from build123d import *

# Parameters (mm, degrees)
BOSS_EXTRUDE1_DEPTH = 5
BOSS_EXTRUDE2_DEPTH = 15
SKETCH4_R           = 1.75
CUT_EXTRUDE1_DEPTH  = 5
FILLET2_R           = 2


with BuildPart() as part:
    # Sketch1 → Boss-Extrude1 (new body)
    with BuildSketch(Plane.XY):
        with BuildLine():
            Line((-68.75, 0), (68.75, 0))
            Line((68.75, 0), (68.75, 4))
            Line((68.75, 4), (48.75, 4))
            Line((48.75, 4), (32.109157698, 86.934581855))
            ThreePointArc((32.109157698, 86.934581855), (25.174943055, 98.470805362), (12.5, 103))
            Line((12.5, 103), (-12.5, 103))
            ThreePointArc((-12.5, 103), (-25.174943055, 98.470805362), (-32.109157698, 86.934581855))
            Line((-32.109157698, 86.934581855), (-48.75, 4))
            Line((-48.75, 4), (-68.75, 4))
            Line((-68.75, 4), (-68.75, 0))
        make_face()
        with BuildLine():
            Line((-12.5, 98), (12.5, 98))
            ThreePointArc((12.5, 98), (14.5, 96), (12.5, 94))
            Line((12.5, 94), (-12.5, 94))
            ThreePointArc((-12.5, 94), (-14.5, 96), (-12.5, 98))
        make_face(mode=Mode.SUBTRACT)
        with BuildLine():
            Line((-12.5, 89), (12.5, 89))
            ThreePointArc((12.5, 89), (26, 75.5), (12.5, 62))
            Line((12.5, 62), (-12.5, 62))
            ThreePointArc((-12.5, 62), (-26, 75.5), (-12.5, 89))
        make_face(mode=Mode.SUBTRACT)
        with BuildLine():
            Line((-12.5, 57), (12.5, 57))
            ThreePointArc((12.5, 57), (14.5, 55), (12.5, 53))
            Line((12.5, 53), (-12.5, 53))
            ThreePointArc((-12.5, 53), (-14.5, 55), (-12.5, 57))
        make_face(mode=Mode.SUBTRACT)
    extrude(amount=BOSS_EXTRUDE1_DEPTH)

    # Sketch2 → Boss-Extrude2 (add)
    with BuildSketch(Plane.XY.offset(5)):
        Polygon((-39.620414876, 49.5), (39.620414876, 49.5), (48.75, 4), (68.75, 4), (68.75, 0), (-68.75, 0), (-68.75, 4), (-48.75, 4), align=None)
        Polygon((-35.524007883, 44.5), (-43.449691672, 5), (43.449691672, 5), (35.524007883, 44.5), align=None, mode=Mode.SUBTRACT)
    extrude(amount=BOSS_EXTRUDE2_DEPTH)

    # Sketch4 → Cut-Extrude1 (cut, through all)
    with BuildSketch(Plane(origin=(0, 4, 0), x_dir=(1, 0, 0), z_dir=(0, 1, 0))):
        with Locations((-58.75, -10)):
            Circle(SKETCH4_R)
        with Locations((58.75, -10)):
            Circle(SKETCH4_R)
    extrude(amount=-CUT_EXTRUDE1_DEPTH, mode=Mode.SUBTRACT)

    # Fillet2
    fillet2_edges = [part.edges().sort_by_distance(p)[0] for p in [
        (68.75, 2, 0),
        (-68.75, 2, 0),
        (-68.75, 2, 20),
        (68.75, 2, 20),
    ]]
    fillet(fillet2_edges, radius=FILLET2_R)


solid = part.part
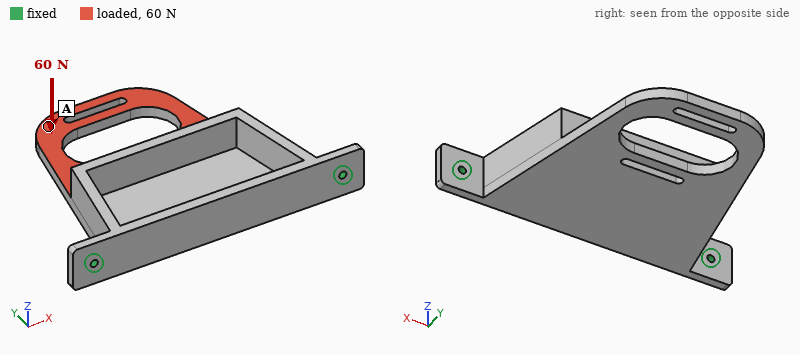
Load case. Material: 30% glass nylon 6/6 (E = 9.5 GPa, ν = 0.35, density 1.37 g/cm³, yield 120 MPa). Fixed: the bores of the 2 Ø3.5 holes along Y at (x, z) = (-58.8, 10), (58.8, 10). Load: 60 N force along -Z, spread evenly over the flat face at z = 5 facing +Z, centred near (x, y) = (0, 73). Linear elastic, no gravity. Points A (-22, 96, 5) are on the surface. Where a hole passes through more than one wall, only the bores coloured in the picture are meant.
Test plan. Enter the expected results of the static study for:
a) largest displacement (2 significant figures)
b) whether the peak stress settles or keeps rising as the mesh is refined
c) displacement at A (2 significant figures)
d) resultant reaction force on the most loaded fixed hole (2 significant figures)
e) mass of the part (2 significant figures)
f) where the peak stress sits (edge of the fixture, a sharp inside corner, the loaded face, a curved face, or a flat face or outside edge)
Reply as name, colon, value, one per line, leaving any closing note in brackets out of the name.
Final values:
largest displacement: 1.9 mm
whether the peak stress settles or keeps rising as the mesh is refined: keeps rising
displacement at A: 1.7 mm
resultant reaction force on the most loaded fixed hole: 31 N
mass of the part: 75 g
where the peak stress sits: edge of the fixture
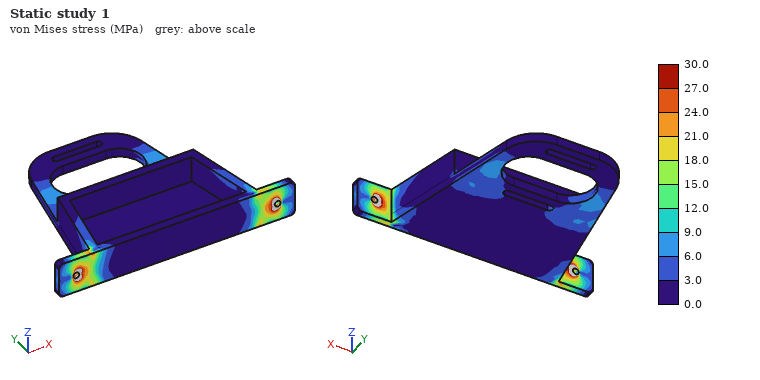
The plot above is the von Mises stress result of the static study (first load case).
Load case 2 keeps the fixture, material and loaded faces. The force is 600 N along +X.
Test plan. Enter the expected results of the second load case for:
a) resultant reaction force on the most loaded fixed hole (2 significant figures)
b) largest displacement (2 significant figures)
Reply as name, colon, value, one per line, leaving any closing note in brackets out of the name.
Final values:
resultant reaction force on the most loaded fixed hole: 500 N
largest displacement: 0.62 mm
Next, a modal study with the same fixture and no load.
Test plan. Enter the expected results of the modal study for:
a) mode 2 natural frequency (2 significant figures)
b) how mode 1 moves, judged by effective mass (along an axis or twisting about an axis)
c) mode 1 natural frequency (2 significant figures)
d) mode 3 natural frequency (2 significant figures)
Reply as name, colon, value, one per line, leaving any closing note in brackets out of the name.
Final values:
mode 2 natural frequency: 820 Hz
how mode 1 moves, judged by effective mass: along Z
mode 1 natural frequency: 230 Hz
mode 3 natural frequency: 840 Hz
